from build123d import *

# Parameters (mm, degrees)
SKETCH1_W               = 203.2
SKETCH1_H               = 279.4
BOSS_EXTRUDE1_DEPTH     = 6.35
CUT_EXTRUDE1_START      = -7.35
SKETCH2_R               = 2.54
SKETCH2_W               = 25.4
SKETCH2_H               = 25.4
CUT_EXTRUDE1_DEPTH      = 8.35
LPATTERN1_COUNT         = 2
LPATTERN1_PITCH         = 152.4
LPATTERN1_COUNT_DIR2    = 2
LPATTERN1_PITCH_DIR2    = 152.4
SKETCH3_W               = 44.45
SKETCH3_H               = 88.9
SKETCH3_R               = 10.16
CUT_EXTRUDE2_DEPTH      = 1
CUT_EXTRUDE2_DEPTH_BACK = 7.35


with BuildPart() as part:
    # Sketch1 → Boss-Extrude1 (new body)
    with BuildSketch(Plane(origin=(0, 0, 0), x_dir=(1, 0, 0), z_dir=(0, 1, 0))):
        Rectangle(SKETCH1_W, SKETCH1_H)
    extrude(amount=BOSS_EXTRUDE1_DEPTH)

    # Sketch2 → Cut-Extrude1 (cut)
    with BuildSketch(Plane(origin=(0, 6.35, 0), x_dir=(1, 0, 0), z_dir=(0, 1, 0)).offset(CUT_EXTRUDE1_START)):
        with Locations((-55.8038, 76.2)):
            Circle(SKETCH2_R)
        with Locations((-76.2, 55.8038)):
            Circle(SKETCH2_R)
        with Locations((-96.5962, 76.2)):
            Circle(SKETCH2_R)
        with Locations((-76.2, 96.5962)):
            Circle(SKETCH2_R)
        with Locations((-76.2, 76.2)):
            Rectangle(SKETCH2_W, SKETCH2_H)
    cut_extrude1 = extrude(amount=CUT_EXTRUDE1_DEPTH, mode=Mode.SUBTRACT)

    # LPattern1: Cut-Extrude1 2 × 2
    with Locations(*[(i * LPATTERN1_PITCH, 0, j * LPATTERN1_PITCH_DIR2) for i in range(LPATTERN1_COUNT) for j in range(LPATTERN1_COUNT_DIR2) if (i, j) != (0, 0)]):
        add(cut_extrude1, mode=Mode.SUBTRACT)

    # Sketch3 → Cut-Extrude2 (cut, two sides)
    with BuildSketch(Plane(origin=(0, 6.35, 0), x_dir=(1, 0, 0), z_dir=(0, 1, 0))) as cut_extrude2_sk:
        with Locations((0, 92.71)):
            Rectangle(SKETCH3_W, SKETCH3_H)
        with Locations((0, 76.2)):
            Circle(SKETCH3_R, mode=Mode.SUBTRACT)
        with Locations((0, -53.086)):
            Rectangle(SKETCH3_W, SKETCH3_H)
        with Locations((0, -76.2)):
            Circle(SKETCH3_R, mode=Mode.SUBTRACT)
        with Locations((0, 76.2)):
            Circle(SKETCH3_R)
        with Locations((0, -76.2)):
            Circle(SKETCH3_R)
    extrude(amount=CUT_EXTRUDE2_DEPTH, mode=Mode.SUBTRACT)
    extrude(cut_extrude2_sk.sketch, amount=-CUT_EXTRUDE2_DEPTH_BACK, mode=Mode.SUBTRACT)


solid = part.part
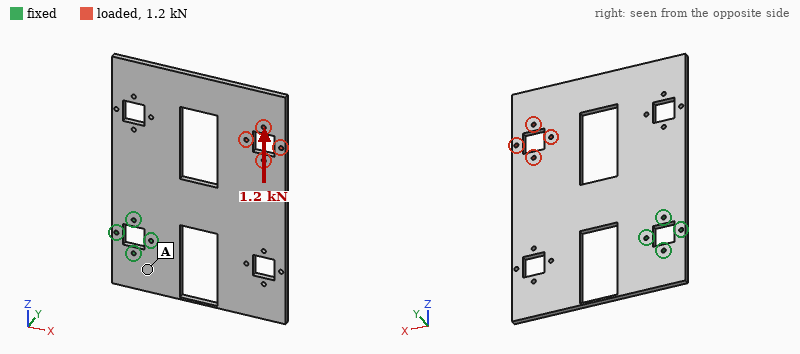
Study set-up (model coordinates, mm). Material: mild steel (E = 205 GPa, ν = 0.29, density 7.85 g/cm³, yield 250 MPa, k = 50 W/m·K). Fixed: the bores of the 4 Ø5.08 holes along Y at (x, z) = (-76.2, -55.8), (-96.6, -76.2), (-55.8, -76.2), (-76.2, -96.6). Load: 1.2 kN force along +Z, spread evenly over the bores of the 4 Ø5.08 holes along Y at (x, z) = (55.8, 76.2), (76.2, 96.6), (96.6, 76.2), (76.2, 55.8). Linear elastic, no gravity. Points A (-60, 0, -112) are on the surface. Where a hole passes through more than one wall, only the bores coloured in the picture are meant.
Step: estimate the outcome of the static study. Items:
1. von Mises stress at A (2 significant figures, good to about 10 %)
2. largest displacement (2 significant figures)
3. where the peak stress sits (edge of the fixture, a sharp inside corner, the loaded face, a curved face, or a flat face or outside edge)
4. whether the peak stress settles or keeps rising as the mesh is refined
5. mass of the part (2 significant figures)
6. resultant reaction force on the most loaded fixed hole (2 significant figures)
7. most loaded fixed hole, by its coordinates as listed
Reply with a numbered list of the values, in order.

1. 4.5 MPa
2. 59 µm
3. edge of the fixture
4. keeps rising
5. 2.3 kg
6. 3.5 kN
7. (-55.8, -76.2)
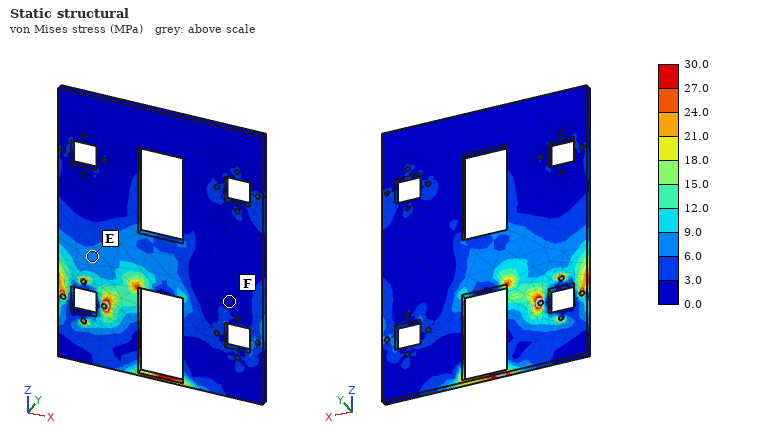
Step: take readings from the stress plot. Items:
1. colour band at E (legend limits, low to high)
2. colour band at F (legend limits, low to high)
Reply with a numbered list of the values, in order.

1. 6.0 to 9.0 MPa
2. 0.0 to 3.0 MPa
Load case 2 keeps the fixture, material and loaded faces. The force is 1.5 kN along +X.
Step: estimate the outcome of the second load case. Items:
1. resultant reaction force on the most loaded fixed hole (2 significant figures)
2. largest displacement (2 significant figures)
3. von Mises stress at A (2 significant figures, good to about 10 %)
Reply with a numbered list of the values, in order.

1. 3.6 kN
2. 69 µm
3. 5.0 MPa
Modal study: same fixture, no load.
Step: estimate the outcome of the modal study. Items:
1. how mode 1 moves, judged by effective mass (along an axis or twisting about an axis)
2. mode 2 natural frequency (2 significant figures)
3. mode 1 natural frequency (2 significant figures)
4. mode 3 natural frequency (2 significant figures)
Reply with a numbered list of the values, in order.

1. along Y
2. 140 Hz
3. 81 Hz
4. 300 Hz
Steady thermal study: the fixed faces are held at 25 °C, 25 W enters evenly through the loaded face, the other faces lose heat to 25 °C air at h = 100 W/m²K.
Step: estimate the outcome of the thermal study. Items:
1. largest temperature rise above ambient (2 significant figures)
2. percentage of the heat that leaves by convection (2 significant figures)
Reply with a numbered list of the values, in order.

1. 28 K
2. 100 %
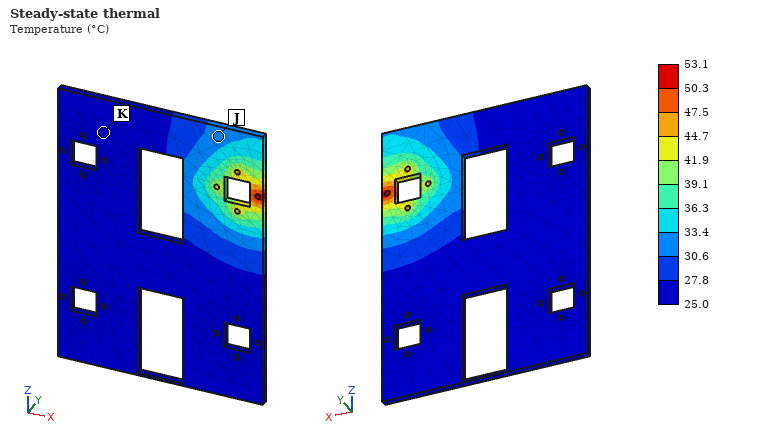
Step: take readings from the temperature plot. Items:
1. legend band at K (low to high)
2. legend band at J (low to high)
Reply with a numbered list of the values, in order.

1. 25.0 to 27.8 °C
2. 30.6 to 33.4 °C
